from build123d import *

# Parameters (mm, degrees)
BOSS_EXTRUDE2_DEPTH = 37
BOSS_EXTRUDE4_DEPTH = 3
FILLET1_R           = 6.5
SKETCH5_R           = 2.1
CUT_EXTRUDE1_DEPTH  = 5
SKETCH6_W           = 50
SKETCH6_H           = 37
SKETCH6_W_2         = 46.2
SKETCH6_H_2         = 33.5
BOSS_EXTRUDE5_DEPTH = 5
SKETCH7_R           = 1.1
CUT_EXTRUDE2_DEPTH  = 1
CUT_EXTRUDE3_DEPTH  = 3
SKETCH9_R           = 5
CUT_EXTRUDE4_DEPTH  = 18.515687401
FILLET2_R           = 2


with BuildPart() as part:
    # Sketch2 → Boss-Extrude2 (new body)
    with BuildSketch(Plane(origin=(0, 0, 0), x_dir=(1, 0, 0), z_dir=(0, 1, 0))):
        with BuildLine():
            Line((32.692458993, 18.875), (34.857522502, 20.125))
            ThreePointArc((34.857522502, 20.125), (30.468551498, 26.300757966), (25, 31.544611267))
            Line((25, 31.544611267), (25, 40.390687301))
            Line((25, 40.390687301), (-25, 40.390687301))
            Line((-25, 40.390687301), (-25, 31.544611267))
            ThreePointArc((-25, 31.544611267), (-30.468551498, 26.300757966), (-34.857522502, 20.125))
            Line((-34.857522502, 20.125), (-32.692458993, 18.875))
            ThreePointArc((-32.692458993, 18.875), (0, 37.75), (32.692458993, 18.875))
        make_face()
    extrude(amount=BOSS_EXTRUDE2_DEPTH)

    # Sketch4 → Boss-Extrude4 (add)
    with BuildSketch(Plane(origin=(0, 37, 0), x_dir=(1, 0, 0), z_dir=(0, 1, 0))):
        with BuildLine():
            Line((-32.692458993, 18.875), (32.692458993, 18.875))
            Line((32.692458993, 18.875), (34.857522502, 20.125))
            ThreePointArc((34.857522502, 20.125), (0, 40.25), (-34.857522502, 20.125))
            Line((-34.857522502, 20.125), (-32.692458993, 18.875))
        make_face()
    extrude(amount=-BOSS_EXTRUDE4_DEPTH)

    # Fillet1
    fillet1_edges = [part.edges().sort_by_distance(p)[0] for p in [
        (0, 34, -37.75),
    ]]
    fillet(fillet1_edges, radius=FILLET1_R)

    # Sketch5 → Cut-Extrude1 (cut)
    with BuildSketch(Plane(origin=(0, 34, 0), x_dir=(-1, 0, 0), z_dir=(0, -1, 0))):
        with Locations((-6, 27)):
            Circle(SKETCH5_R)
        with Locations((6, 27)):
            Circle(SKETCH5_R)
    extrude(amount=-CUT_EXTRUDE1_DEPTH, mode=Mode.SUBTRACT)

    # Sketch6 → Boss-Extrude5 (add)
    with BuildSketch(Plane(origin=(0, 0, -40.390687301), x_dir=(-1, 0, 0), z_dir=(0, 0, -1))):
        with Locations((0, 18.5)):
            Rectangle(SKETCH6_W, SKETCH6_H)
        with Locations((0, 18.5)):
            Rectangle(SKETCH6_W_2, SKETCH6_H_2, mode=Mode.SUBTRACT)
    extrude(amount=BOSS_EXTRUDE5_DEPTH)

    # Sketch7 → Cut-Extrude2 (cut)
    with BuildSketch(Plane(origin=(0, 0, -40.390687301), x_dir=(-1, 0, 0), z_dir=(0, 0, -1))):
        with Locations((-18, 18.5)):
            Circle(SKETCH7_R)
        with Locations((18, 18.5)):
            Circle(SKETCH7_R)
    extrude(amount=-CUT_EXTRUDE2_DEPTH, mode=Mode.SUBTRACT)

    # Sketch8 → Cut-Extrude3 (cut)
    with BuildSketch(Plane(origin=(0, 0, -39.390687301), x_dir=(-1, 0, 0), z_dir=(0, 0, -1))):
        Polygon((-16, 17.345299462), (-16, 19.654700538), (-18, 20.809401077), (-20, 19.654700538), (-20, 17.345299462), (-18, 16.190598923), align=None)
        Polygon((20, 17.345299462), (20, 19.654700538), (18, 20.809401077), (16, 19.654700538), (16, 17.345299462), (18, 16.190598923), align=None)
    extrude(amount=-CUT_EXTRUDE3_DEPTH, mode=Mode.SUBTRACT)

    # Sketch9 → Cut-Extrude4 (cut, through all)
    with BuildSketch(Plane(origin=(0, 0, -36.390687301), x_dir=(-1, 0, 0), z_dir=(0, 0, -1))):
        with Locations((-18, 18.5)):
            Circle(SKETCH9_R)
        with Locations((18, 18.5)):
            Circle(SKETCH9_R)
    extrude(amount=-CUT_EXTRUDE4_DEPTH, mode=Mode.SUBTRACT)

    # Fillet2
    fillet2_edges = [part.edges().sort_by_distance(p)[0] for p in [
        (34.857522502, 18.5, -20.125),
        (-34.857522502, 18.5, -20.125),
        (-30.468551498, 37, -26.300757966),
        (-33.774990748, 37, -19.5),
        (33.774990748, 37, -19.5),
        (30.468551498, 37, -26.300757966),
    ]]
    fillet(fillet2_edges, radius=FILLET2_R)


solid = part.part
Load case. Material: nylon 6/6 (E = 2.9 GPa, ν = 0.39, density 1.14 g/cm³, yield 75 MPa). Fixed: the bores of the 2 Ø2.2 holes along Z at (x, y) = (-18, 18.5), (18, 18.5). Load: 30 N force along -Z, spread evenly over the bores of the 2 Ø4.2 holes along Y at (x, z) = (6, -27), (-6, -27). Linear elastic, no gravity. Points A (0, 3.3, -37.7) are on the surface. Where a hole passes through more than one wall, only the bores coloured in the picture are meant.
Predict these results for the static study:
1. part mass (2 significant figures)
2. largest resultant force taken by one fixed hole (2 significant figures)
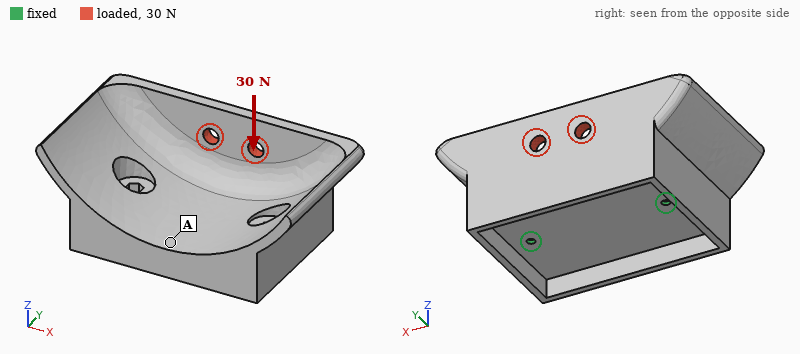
19 g
15 N
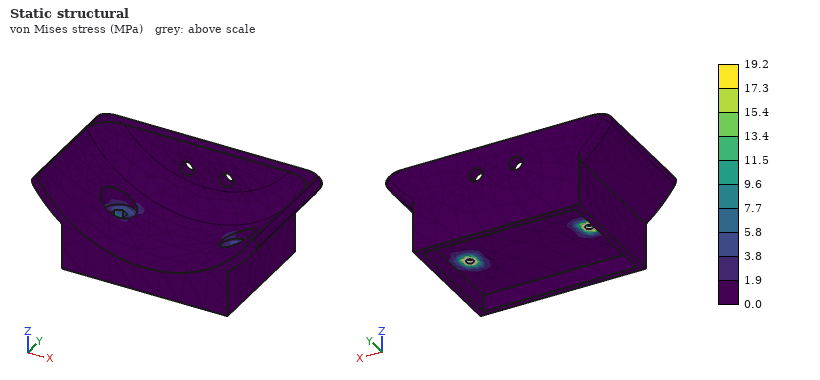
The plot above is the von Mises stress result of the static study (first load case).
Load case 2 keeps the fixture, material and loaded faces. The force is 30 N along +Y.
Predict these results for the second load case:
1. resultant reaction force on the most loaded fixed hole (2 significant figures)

16 N
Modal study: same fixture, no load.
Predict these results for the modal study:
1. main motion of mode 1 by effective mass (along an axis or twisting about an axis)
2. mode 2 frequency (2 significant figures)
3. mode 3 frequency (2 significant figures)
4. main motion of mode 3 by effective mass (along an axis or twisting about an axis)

along Y
1200 Hz
1900 Hz
along X
